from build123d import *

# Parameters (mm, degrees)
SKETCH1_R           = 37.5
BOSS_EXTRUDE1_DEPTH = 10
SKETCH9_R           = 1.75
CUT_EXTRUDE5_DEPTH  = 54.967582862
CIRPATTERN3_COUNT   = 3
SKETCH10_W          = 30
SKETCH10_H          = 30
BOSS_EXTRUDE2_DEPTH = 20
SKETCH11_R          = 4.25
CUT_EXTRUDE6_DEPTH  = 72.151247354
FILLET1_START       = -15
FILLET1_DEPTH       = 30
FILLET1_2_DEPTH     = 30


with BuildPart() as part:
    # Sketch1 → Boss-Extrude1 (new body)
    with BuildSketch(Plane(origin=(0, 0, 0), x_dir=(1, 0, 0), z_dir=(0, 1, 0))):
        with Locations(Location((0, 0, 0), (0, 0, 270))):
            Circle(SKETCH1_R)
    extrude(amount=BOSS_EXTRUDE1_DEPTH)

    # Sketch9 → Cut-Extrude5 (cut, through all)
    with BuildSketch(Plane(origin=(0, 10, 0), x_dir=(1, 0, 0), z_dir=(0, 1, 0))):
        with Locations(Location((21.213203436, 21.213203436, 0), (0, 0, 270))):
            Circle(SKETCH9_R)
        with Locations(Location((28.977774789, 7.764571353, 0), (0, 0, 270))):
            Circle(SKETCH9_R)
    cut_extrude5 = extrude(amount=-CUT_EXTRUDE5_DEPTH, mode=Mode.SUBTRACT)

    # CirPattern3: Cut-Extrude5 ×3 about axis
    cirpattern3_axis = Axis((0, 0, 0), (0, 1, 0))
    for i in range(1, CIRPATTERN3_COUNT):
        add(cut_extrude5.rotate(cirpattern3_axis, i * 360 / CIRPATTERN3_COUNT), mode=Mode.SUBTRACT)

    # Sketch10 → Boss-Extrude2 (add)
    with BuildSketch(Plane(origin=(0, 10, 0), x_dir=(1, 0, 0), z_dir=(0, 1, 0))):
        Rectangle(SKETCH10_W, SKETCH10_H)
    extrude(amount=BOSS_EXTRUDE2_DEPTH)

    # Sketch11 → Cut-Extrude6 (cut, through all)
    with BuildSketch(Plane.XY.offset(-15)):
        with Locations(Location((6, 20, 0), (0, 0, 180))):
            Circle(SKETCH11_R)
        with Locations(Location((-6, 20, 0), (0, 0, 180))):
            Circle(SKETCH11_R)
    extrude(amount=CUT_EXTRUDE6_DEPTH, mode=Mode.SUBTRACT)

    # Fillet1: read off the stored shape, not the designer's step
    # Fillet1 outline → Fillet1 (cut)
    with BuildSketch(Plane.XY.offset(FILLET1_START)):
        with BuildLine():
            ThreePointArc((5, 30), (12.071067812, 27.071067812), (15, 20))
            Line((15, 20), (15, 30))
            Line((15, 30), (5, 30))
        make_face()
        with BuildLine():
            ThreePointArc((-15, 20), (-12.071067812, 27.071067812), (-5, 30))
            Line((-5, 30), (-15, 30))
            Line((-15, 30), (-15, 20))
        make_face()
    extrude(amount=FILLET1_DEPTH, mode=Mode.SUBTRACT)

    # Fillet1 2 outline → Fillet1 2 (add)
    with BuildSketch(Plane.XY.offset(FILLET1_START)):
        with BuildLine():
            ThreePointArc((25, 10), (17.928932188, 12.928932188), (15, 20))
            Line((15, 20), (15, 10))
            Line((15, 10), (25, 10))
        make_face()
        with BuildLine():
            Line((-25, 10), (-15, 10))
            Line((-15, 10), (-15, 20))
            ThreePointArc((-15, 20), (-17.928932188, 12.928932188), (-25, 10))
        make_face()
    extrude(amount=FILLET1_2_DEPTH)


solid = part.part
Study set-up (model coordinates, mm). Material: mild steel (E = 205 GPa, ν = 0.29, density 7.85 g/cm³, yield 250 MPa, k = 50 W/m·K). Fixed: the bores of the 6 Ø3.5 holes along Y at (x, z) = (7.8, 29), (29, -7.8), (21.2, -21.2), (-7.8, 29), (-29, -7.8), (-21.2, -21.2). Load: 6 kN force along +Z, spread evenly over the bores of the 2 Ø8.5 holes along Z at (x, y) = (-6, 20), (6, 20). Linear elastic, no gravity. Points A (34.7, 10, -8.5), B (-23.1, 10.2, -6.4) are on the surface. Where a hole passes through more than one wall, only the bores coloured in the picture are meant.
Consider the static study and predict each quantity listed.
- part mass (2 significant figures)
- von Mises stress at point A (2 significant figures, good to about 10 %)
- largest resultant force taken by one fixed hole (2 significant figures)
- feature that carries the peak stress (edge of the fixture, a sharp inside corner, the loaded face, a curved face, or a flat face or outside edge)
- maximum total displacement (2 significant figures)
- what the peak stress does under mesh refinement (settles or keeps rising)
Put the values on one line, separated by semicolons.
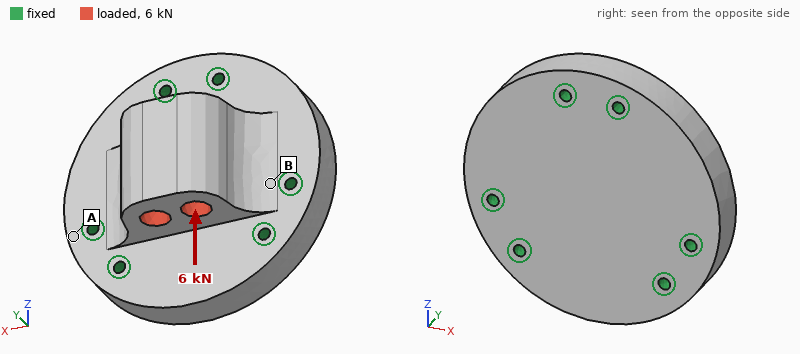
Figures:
460 g; 4.4 MPa; 1.6 kN; edge of the fixture; 5.8 µm; keeps rising
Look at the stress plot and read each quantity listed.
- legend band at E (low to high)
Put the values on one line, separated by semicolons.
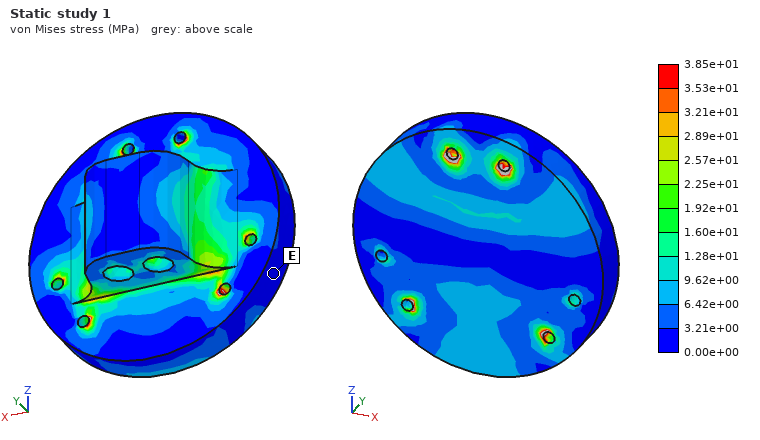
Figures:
0.00e+00 to 3.21e+00 MPa
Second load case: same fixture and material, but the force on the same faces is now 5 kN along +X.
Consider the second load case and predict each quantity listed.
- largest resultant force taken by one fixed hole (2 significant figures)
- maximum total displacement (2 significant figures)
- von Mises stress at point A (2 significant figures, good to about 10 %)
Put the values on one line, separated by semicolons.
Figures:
1.5 kN; 3.8 µm; 3.6 MPa
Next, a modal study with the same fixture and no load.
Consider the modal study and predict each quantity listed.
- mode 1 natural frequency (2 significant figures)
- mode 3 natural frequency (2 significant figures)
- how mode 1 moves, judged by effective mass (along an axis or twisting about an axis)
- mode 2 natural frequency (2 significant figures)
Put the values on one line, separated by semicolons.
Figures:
14 kHz; 16 kHz; along Y; 16 kHz
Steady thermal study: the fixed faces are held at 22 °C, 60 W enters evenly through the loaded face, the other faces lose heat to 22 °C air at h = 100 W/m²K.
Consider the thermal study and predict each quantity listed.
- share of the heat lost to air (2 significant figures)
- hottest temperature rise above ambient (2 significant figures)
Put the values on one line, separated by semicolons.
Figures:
22 %; 36 K
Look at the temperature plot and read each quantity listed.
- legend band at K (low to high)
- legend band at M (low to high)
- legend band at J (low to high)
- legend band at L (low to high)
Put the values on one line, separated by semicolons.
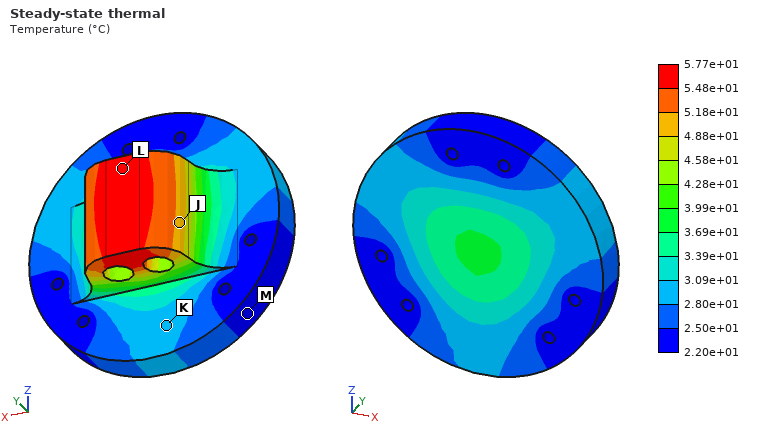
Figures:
2.80e+01 to 3.09e+01 °C; 2.20e+01 to 2.50e+01 °C; 4.88e+01 to 5.18e+01 °C; 5.48e+01 to 5.77e+01 °C
